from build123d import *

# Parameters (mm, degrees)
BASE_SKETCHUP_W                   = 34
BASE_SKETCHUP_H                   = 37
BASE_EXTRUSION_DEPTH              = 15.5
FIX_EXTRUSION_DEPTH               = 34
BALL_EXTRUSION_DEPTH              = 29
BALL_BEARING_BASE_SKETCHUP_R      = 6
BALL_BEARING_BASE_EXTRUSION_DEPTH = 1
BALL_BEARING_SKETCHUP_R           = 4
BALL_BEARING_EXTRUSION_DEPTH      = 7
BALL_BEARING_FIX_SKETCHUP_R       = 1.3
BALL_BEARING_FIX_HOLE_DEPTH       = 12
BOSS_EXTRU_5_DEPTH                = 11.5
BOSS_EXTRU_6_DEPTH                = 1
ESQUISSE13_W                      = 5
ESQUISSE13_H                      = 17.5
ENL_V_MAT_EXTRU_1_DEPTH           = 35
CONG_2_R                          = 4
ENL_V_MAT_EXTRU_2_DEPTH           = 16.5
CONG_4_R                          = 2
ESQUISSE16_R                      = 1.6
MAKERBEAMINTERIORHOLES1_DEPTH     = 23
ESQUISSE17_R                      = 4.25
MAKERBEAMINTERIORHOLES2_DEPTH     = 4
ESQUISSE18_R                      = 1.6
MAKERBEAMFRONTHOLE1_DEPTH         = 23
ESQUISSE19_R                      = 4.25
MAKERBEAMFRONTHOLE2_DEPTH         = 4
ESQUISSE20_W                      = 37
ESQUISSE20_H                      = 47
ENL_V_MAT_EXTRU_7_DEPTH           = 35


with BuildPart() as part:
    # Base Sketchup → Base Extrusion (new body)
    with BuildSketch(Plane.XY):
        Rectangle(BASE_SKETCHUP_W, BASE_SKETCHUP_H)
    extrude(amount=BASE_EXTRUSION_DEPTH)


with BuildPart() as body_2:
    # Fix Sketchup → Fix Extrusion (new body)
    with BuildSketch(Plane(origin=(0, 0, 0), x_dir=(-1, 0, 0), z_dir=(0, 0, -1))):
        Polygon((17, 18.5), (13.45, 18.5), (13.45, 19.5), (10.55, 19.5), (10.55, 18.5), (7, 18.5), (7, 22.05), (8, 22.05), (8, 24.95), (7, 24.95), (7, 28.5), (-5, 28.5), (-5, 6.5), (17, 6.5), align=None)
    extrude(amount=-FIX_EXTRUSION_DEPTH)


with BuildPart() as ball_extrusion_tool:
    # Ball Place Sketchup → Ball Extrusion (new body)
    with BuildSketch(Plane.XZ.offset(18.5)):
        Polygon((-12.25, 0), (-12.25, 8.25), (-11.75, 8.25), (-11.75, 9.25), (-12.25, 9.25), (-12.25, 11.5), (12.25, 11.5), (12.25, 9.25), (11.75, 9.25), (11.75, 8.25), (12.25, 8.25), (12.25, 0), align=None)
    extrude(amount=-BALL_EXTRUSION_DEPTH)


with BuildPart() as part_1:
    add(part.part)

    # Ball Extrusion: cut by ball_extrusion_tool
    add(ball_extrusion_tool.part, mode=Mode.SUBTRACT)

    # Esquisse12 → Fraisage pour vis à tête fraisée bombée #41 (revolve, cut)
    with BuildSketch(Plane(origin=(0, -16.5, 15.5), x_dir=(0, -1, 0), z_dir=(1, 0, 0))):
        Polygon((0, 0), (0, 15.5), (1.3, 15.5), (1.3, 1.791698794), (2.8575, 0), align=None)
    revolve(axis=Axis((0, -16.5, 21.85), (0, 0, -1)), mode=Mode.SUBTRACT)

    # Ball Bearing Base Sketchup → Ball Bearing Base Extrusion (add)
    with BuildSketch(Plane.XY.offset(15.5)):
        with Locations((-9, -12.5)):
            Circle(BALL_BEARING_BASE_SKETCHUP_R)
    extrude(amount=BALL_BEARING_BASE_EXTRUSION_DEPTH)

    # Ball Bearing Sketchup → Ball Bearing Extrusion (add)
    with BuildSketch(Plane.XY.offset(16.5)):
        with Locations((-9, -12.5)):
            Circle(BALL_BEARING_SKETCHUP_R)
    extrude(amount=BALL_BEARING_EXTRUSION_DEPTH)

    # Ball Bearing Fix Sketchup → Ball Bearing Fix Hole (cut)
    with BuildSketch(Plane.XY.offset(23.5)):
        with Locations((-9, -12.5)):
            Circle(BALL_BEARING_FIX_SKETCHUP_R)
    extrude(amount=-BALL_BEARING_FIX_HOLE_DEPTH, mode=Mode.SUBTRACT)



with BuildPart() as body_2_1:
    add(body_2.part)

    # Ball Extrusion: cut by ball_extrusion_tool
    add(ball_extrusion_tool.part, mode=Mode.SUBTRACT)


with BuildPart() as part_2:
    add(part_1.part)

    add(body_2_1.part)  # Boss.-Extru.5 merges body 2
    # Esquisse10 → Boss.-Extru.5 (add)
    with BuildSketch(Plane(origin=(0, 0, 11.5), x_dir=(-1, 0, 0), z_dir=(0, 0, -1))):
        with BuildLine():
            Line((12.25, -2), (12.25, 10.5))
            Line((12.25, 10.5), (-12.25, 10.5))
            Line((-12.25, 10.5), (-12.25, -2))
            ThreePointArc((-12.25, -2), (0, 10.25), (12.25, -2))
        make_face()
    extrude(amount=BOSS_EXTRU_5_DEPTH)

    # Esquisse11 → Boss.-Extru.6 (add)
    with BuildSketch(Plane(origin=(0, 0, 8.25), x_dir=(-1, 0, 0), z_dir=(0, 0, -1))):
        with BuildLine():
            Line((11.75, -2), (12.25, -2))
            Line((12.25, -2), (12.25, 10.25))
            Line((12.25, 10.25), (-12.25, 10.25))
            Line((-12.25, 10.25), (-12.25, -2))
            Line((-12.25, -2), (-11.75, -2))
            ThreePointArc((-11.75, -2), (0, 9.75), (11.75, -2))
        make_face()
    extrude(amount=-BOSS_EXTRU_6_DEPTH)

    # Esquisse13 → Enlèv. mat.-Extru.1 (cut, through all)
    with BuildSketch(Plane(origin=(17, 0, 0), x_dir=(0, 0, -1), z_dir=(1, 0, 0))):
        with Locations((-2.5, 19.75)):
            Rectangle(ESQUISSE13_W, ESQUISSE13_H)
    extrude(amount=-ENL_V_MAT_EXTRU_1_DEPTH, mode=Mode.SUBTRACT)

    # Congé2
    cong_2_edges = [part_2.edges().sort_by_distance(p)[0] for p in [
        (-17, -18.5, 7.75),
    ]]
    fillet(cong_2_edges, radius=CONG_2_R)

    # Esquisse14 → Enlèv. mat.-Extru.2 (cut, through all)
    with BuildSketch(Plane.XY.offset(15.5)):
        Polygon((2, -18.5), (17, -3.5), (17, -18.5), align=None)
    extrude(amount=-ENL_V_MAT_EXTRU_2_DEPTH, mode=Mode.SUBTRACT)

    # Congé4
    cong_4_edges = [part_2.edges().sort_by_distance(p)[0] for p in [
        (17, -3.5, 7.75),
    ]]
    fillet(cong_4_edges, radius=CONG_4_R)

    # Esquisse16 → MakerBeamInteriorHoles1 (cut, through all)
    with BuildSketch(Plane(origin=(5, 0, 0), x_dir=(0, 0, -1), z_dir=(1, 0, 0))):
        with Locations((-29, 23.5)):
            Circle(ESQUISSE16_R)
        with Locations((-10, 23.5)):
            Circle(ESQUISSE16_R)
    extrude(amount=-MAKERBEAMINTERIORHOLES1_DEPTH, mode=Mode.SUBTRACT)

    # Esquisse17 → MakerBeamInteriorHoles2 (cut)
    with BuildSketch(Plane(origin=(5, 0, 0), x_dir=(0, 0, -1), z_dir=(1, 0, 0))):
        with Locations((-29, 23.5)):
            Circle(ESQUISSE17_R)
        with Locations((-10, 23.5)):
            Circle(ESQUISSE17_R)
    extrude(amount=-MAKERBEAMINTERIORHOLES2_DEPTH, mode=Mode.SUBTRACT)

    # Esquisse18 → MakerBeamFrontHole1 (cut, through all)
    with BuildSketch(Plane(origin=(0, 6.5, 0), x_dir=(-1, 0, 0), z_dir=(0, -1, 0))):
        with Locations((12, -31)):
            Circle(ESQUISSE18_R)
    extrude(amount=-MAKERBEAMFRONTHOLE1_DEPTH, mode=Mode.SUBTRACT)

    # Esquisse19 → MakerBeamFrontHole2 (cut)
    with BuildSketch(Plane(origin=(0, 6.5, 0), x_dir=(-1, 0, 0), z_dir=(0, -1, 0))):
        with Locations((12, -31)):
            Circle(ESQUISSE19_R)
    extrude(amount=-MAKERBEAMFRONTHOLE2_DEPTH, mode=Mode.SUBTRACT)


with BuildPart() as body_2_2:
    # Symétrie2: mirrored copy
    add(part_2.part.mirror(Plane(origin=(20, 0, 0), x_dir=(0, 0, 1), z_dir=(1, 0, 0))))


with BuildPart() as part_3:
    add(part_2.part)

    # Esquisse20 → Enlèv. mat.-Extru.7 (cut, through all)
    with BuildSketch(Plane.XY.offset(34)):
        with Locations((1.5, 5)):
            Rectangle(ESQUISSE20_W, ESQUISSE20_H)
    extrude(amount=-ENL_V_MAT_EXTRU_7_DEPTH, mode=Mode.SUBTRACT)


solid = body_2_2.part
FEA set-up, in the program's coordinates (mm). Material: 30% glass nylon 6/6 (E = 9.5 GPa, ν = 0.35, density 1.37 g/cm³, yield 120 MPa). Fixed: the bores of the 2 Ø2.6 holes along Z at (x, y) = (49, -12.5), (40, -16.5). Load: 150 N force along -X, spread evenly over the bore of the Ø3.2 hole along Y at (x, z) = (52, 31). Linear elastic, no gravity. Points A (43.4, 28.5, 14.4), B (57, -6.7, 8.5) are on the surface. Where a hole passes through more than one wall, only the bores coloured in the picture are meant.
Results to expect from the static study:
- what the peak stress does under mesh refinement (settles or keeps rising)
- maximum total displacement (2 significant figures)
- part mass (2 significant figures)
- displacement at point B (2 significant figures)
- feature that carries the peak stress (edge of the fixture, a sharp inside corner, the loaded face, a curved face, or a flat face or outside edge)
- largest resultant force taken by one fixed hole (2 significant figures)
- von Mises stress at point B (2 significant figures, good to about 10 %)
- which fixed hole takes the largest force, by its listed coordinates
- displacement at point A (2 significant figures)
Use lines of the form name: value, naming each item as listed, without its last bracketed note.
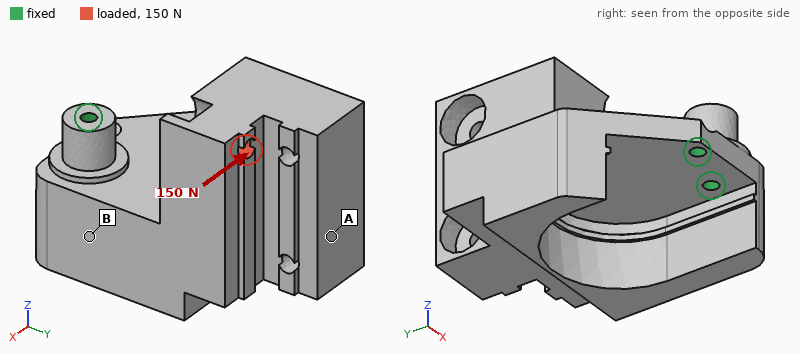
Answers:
what the peak stress does under mesh refinement: keeps rising
maximum total displacement: 0.28 mm
part mass: 24 g
displacement at point B: 0.047 mm
feature that carries the peak stress: edge of the fixture
largest resultant force taken by one fixed hole: 420 N
von Mises stress at point B: 10 MPa
which fixed hole takes the largest force, by its listed coordinates: (49, -12.5)
displacement at point A: 0.099 mm
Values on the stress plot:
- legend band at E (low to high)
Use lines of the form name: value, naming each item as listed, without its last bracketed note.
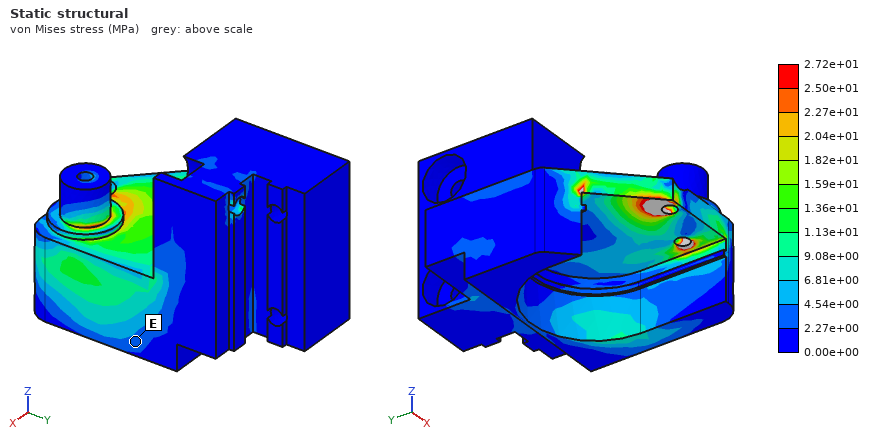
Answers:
legend band at E: 2.27e+00 to 4.54e+00 MPa
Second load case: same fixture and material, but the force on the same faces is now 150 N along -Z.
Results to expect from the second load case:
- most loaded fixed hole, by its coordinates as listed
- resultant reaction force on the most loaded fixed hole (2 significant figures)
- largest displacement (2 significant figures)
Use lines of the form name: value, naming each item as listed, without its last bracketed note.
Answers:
most loaded fixed hole, by its coordinates as listed: (49, -12.5)
resultant reaction force on the most loaded fixed hole: 220 N
largest displacement: 0.42 mm
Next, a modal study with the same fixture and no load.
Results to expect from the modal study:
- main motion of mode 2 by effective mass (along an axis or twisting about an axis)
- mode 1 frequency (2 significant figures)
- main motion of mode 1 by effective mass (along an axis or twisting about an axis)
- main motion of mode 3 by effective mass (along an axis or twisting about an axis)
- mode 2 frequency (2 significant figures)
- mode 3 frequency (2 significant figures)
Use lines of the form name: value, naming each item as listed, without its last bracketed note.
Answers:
main motion of mode 2 by effective mass: along X
mode 1 frequency: 830 Hz
main motion of mode 1 by effective mass: along Z
main motion of mode 3 by effective mass: along X
mode 2 frequency: 1500 Hz
mode 3 frequency: 1700 Hz
